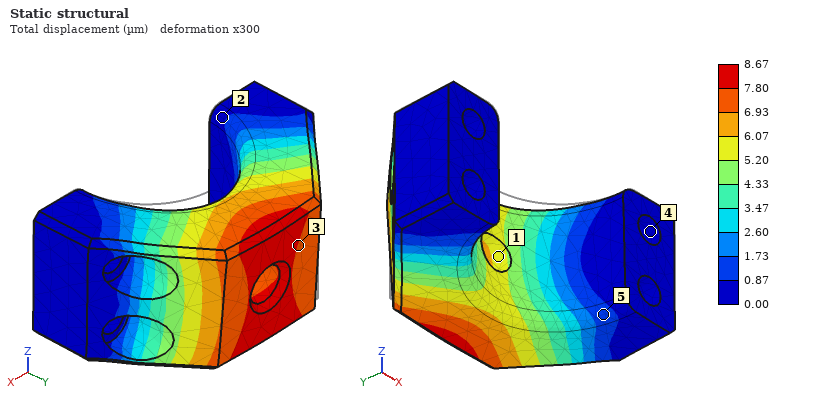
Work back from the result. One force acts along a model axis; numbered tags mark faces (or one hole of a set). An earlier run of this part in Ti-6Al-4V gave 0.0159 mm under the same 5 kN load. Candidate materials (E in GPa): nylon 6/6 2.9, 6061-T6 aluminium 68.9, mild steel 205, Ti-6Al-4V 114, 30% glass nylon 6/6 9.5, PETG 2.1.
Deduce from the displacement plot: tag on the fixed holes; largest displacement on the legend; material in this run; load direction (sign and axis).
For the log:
4
8.67 µm
mild steel
-Z
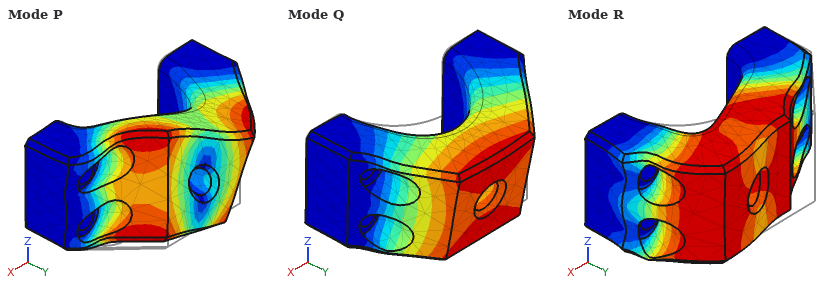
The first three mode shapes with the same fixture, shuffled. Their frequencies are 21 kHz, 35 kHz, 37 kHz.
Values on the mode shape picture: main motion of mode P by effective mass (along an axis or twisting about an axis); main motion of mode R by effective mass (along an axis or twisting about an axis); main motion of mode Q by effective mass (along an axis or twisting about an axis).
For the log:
twisting about Y
along X
along Z
